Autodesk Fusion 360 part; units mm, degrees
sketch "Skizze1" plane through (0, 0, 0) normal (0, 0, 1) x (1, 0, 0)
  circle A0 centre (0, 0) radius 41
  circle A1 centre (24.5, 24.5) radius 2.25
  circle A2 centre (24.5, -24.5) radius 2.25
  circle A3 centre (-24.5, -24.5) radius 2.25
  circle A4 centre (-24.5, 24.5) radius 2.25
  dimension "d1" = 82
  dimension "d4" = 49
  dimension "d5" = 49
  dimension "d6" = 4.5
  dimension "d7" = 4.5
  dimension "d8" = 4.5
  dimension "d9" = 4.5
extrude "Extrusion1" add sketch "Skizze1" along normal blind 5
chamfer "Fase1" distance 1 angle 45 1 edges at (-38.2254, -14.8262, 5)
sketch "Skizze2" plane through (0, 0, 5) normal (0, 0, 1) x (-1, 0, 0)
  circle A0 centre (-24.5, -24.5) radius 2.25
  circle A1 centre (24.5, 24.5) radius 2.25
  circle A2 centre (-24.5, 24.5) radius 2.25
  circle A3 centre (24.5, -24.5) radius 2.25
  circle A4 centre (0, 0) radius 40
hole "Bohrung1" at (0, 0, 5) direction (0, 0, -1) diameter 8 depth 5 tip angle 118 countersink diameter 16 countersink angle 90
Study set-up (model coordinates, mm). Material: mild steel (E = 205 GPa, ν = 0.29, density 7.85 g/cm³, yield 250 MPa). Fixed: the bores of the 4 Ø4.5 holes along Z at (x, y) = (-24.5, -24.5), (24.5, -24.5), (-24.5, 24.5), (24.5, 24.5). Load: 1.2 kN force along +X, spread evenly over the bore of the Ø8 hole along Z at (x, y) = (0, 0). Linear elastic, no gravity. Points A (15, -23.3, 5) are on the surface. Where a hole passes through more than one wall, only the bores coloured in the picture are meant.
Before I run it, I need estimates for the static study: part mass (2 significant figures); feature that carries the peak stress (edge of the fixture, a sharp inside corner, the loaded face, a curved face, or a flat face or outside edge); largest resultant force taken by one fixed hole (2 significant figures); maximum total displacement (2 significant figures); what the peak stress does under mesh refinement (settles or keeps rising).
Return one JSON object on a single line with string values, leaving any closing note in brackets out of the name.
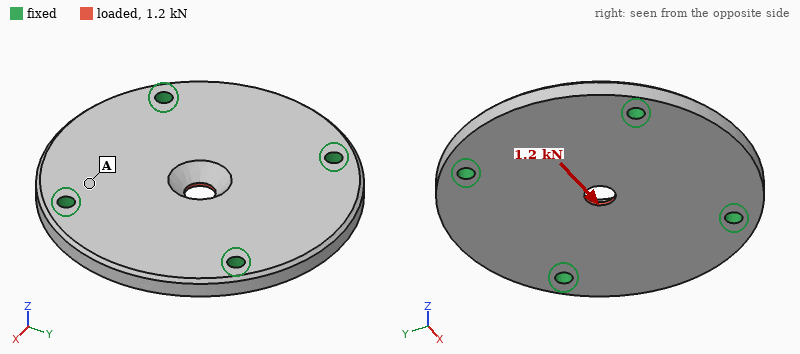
{"part mass": "200 g", "feature that carries the peak stress": "a sharp inside corner", "largest resultant force taken by one fixed hole": "310 N", "maximum total displacement": "1.8 µm", "what the peak stress does under mesh refinement": "keeps rising"}
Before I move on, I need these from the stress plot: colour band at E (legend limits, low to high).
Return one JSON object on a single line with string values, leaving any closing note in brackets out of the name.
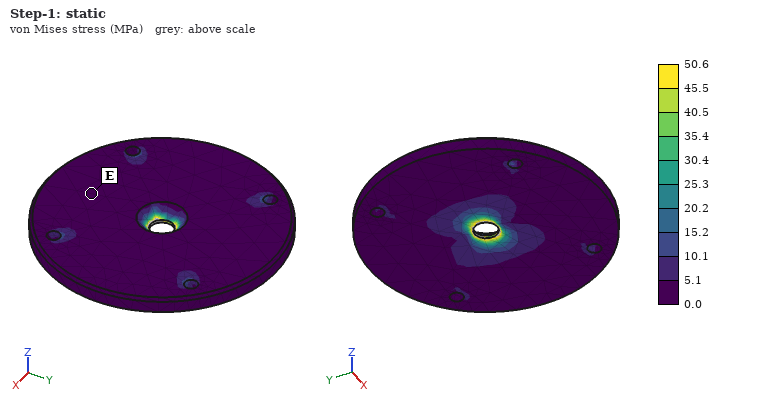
{"colour band at E": "0.0 to 5.1 MPa"}
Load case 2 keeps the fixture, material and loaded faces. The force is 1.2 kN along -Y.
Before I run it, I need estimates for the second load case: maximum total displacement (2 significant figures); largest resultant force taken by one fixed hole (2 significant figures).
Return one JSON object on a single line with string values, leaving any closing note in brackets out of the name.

{"maximum total displacement": "1.8 µm", "largest resultant force taken by one fixed hole": "310 N"}
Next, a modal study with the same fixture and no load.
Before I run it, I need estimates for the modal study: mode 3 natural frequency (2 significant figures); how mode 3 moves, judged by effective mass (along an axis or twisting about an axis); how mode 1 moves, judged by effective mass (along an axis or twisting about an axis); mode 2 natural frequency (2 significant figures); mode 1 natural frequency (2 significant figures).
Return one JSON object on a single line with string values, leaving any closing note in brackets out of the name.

{"mode 3 natural frequency": "8800 Hz", "how mode 3 moves, judged by effective mass": "twisting about Y", "how mode 1 moves, judged by effective mass": "along Z", "mode 2 natural frequency": "8300 Hz", "mode 1 natural frequency": "7500 Hz"}
